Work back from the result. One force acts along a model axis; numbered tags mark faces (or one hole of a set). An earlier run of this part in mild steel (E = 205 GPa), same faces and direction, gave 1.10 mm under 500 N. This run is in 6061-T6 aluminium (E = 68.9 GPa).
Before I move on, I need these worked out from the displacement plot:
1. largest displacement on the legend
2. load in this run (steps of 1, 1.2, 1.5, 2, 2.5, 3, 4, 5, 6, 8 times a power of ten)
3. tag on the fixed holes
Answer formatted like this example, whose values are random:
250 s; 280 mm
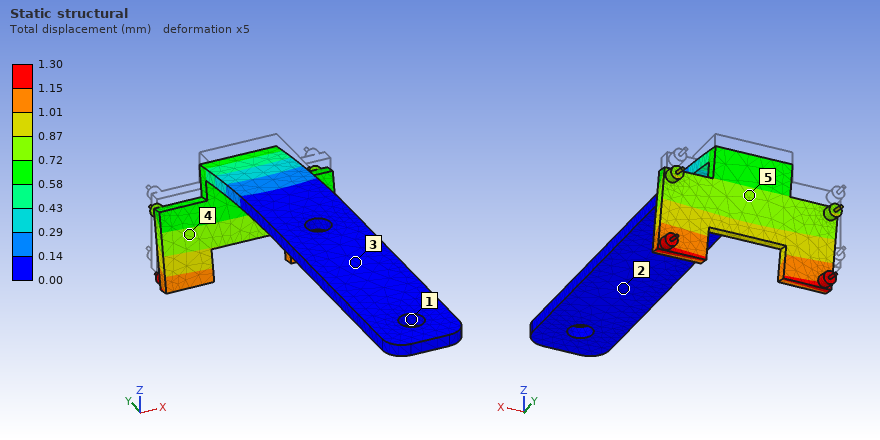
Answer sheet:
1.30 mm; 200 N; 1
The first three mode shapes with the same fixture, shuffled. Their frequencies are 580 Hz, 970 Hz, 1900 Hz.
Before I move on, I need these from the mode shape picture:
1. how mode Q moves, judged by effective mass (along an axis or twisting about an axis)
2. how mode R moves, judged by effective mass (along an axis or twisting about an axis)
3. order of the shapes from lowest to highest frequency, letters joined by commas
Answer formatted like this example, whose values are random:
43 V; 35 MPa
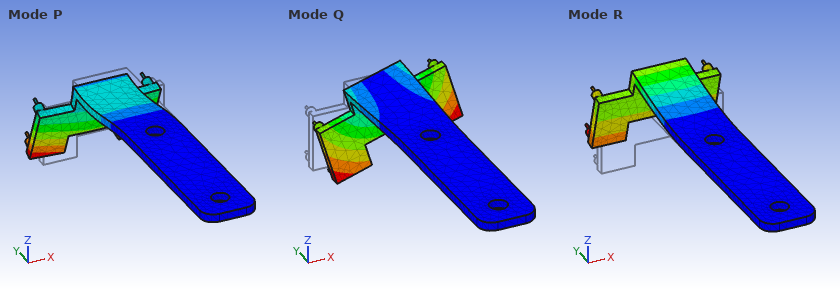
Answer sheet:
along X; along Z; R, Q, P
